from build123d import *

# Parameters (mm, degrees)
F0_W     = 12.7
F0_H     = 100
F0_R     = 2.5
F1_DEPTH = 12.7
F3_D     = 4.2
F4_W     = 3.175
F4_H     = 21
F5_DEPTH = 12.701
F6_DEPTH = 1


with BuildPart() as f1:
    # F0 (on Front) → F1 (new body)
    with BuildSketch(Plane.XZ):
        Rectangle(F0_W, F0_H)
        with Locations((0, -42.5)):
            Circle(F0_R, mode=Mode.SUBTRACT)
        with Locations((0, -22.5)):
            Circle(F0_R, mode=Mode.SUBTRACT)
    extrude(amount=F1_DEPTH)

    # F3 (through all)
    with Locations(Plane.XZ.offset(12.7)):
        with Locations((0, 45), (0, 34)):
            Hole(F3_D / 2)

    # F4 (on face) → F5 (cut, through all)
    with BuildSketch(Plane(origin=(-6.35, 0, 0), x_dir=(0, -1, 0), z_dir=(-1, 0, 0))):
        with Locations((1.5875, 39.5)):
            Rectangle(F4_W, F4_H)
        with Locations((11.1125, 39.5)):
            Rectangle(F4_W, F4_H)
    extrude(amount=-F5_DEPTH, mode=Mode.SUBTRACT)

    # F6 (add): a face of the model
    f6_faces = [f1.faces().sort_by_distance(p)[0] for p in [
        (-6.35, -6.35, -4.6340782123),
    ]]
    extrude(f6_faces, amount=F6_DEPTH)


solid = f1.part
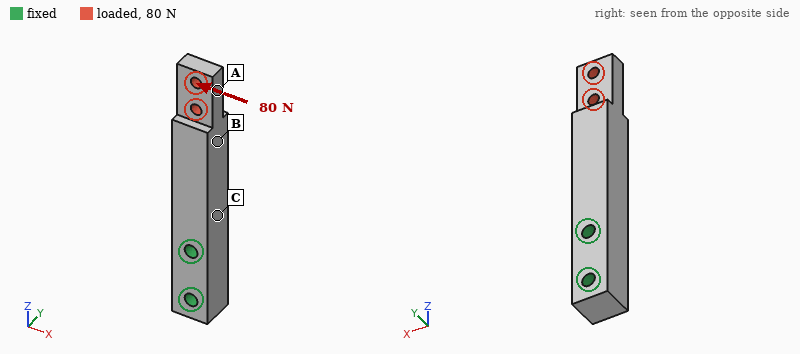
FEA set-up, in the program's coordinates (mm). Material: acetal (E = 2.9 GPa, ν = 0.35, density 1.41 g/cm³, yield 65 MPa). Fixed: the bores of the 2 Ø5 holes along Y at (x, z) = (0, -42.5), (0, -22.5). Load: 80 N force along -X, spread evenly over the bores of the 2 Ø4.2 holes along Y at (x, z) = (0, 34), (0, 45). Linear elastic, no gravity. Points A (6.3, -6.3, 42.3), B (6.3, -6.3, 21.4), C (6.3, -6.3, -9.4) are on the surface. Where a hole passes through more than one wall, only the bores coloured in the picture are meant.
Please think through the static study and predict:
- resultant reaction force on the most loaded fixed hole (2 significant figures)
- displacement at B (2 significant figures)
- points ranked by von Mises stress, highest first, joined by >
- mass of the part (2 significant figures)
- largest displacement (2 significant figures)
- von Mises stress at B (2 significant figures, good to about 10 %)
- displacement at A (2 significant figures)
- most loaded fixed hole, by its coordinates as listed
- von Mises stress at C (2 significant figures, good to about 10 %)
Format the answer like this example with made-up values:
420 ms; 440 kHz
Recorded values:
180 N; 0.58 mm; C > B > A; 21 g; 1.2 mm; 4.0 MPa; 1.0 mm; (0, -22.5); 9.9 MPa
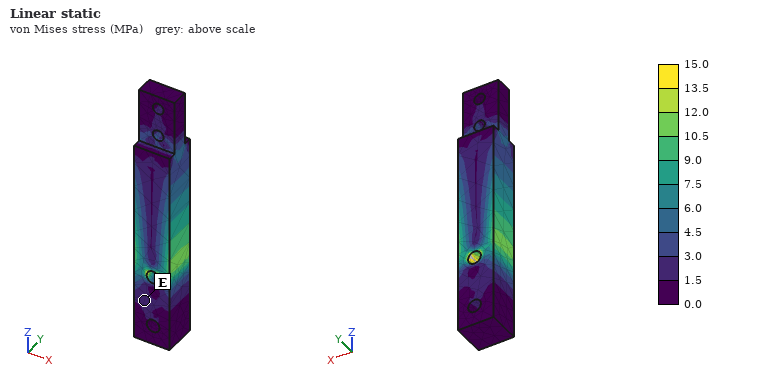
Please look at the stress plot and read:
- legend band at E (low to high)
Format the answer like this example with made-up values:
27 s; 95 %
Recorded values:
1.5 to 3.0 MPa
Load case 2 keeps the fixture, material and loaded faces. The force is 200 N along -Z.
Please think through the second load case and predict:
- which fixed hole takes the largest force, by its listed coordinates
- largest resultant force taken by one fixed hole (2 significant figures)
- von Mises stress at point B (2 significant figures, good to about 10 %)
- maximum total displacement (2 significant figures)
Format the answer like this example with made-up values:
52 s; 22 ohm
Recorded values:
(0, -22.5); 190 N; 1.8 MPa; 49 µm
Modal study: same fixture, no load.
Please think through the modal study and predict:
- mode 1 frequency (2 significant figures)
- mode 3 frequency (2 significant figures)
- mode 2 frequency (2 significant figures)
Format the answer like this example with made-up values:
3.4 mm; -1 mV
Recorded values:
700 Hz; 2800 Hz; 710 Hz
